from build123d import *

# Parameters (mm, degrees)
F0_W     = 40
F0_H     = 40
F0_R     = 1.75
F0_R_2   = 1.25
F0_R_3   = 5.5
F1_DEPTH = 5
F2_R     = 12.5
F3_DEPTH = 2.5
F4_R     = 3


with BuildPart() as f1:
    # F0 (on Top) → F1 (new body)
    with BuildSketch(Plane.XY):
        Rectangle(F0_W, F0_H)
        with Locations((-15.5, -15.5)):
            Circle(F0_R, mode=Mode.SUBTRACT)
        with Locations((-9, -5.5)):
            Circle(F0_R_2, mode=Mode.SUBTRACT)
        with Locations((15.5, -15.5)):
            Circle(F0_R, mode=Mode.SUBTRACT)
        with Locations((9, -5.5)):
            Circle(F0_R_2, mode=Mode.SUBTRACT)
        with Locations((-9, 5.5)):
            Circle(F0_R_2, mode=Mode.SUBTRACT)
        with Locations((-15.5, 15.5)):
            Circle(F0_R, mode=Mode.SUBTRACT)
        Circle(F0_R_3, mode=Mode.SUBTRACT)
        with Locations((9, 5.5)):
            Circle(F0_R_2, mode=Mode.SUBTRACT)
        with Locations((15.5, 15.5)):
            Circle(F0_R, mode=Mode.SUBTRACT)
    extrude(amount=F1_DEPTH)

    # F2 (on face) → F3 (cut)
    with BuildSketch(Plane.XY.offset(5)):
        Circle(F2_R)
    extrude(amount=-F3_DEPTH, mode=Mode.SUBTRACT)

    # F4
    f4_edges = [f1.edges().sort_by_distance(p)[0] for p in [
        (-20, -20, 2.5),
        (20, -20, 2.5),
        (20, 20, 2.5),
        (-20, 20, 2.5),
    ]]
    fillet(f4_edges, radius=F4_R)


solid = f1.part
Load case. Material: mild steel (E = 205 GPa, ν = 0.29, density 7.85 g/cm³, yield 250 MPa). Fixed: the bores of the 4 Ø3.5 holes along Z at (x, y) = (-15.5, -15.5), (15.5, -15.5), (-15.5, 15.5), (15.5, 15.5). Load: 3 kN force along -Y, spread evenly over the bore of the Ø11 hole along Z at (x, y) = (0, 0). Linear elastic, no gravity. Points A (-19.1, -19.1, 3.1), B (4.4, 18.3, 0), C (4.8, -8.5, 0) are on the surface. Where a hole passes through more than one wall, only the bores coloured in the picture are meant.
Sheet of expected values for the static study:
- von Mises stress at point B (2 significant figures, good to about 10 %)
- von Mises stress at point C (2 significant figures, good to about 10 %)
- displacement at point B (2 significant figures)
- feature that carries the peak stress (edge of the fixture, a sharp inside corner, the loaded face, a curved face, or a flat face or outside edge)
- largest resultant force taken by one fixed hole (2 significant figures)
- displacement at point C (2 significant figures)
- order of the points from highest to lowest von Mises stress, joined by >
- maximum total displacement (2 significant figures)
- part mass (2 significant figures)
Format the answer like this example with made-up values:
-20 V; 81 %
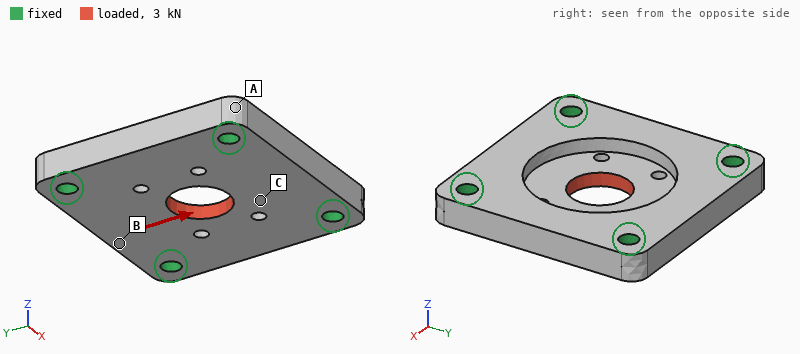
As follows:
11 MPa; 24 MPa; 1.8 µm; a curved face; 820 N; 2.3 µm; C > B > A; 3.2 µm; 49 g
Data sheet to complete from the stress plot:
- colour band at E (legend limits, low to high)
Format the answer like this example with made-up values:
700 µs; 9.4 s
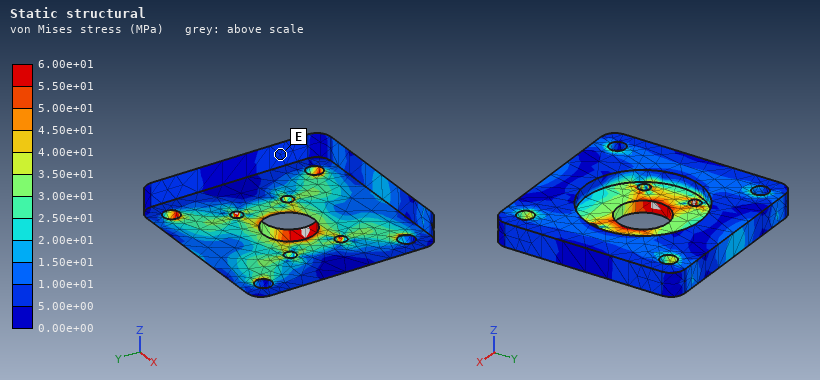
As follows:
5.00e+00 to 1.00e+01 MPa
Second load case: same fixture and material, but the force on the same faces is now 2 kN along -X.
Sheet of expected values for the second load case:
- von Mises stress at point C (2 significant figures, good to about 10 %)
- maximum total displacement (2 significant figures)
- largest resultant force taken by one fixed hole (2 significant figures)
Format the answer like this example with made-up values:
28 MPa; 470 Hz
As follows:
16 MPa; 2.2 µm; 550 N
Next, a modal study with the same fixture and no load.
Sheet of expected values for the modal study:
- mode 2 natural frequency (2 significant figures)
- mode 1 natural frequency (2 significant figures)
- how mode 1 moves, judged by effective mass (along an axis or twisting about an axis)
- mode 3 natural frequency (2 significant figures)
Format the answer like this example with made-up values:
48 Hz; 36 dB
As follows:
25 kHz; 20 kHz; along Z; 25 kHz
